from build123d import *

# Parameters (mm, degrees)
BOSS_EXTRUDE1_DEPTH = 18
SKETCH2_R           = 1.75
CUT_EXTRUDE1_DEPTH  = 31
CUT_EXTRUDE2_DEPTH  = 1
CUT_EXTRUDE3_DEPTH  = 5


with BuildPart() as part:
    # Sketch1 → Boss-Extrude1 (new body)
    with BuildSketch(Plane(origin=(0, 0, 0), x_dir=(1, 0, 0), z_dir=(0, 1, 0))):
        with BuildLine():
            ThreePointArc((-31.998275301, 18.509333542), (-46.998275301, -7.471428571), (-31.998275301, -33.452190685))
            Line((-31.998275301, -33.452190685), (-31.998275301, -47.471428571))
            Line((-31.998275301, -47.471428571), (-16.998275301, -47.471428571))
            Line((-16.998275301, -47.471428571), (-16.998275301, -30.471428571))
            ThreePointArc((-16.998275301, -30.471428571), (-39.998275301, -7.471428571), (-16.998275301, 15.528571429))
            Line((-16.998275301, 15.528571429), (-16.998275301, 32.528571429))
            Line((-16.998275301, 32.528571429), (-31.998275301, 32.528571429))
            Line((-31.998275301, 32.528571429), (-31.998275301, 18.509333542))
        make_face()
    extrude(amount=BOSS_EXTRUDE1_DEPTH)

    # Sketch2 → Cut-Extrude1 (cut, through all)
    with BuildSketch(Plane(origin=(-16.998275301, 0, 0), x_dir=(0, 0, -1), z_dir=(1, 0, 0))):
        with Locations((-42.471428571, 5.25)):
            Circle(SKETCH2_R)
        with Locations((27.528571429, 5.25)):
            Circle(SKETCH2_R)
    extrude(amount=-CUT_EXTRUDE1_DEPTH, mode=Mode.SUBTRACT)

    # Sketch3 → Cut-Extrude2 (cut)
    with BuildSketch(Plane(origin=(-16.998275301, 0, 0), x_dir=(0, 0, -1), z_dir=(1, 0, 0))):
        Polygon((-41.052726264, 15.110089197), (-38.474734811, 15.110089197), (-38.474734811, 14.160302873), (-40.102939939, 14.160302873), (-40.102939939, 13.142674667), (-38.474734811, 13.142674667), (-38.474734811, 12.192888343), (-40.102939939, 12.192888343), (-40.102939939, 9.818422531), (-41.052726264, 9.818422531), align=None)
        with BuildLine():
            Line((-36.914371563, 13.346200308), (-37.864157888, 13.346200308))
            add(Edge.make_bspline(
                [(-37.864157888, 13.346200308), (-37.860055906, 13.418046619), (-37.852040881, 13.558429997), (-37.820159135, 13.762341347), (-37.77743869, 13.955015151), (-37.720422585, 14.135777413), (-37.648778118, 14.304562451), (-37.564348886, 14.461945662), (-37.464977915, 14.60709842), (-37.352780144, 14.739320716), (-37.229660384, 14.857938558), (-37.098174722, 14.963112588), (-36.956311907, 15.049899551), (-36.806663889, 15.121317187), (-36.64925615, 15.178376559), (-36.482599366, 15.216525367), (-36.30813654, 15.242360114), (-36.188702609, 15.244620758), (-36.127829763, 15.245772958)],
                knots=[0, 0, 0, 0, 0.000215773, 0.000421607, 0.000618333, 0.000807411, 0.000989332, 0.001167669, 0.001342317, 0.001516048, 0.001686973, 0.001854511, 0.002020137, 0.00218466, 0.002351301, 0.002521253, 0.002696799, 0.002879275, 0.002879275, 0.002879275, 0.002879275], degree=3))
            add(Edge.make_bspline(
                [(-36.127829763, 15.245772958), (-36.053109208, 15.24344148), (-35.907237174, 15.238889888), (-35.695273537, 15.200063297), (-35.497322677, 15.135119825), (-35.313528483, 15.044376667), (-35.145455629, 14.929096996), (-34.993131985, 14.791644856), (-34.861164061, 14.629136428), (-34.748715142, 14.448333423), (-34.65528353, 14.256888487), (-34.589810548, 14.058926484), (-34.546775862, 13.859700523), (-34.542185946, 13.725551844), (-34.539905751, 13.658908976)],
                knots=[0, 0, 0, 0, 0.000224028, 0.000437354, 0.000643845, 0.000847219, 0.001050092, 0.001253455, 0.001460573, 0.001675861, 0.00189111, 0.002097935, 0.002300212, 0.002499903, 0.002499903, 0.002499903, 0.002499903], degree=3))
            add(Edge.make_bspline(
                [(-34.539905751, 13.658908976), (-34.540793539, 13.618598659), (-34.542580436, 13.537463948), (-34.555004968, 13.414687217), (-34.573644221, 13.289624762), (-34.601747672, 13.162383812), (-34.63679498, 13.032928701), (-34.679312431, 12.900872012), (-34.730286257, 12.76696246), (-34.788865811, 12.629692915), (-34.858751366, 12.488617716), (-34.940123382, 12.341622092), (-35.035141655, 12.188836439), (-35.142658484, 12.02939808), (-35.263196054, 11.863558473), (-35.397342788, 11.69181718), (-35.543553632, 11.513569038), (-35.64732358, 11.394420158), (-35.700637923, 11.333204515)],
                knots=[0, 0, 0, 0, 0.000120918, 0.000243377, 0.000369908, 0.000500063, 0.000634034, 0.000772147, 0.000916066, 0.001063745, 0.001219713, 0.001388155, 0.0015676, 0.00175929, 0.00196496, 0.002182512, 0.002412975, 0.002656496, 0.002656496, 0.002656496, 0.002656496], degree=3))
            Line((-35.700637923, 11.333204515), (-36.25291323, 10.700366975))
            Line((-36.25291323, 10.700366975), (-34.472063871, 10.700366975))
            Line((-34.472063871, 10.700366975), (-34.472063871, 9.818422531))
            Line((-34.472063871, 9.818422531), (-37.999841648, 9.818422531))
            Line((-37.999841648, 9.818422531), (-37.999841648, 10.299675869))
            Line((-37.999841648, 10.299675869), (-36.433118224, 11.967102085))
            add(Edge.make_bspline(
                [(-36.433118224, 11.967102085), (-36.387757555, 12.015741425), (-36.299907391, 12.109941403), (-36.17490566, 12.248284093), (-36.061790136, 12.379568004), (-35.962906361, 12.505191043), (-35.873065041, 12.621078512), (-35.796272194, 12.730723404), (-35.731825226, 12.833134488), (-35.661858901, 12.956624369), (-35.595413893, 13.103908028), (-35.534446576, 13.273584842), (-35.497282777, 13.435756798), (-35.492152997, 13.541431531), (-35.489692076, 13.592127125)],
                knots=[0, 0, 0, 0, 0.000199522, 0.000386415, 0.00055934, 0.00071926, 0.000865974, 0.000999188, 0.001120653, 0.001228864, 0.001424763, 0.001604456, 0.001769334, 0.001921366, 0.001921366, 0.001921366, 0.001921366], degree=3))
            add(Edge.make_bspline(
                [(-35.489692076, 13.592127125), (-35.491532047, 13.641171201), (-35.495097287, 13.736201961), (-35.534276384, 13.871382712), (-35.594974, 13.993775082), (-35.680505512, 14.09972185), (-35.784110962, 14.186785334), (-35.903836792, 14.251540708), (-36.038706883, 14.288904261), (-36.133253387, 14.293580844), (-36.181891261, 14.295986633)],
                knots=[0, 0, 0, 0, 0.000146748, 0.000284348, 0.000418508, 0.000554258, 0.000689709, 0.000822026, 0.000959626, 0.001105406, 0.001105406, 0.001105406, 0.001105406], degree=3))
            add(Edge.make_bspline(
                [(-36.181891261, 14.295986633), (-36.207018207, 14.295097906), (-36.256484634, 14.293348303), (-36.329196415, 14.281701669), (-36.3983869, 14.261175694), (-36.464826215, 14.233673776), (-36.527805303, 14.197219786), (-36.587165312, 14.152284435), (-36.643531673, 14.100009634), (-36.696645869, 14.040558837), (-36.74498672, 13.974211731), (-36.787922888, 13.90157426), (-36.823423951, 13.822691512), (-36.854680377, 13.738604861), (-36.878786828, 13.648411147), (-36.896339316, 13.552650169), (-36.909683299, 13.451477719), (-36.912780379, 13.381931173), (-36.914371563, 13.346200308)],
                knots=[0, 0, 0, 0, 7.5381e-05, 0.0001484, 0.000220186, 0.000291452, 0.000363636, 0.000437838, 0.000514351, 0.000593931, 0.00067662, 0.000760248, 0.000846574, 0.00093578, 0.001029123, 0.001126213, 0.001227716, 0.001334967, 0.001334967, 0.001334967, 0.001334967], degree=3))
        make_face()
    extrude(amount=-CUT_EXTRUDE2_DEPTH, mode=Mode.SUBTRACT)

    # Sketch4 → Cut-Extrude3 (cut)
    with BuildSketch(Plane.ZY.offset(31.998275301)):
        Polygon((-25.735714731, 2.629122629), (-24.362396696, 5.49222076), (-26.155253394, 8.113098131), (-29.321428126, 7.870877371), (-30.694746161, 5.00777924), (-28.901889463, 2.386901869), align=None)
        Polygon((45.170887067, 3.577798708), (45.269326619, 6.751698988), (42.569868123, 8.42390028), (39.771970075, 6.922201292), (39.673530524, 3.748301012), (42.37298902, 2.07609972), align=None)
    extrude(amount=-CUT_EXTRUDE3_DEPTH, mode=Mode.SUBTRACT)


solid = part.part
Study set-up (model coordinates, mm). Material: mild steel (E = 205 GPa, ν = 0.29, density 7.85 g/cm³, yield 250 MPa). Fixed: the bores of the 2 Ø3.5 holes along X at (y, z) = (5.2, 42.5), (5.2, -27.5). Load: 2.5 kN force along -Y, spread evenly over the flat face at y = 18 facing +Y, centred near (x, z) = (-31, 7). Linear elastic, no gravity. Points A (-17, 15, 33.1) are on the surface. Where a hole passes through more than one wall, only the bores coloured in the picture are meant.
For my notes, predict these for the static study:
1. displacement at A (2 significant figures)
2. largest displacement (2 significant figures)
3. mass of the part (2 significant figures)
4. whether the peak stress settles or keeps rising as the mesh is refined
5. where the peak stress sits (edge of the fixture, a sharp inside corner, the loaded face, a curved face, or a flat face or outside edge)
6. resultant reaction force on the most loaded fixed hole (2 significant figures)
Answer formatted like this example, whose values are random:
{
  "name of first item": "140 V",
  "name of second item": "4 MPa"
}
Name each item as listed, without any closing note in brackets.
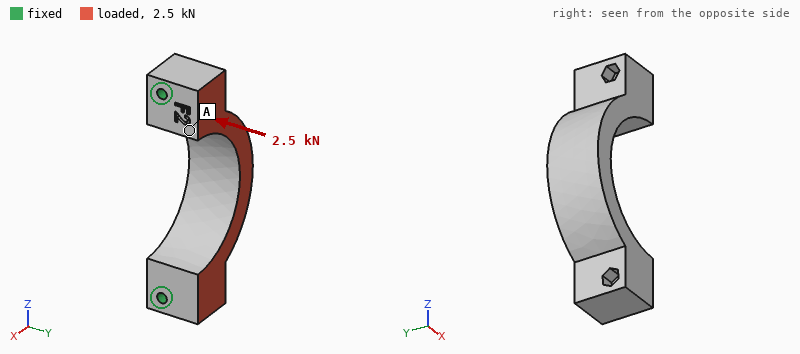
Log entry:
{
  "displacement at A": "4.7 µm",
  "largest displacement": "20 µm",
  "mass of the part": "130 g",
  "whether the peak stress settles or keeps rising as the mesh is refined": "keeps rising",
  "where the peak stress sits": "edge of the fixture",
  "resultant reaction force on the most loaded fixed hole": "1.3 kN"
}
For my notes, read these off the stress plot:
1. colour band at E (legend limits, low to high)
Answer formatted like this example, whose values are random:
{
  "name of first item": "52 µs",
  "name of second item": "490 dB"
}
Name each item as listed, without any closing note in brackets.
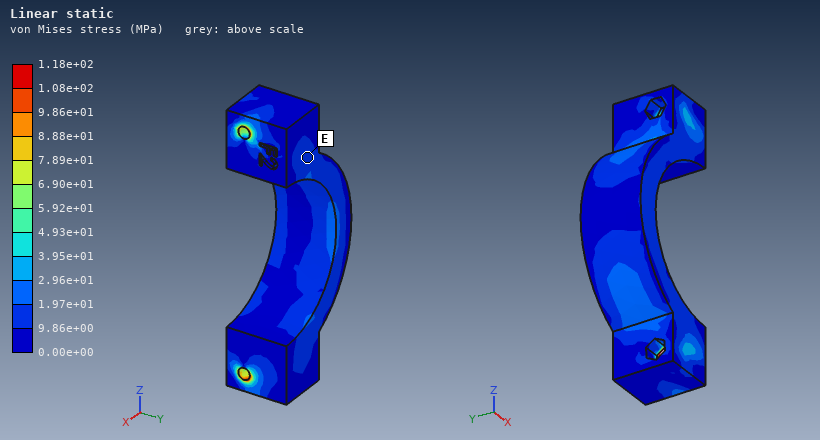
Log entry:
{
  "colour band at E": "9.86e+00 to 1.97e+01 MPa"
}
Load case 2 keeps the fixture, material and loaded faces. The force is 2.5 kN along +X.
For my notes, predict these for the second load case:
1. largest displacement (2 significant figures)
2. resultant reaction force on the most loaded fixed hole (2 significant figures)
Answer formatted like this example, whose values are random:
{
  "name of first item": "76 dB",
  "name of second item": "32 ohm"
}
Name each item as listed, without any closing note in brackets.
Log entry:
{
  "largest displacement": "17 µm",
  "resultant reaction force on the most loaded fixed hole": "1.3 kN"
}
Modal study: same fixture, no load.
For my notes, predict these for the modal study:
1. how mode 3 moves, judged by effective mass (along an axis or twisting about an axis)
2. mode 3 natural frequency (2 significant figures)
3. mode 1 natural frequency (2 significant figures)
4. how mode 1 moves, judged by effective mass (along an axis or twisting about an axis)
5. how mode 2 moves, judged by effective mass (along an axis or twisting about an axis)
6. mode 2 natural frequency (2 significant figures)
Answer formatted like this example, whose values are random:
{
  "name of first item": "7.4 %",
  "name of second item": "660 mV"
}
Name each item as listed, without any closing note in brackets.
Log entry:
{
  "how mode 3 moves, judged by effective mass": "along X",
  "mode 3 natural frequency": "17 kHz",
  "mode 1 natural frequency": "6100 Hz",
  "how mode 1 moves, judged by effective mass": "along Y",
  "how mode 2 moves, judged by effective mass": "along Z",
  "mode 2 natural frequency": "13 kHz"
}
